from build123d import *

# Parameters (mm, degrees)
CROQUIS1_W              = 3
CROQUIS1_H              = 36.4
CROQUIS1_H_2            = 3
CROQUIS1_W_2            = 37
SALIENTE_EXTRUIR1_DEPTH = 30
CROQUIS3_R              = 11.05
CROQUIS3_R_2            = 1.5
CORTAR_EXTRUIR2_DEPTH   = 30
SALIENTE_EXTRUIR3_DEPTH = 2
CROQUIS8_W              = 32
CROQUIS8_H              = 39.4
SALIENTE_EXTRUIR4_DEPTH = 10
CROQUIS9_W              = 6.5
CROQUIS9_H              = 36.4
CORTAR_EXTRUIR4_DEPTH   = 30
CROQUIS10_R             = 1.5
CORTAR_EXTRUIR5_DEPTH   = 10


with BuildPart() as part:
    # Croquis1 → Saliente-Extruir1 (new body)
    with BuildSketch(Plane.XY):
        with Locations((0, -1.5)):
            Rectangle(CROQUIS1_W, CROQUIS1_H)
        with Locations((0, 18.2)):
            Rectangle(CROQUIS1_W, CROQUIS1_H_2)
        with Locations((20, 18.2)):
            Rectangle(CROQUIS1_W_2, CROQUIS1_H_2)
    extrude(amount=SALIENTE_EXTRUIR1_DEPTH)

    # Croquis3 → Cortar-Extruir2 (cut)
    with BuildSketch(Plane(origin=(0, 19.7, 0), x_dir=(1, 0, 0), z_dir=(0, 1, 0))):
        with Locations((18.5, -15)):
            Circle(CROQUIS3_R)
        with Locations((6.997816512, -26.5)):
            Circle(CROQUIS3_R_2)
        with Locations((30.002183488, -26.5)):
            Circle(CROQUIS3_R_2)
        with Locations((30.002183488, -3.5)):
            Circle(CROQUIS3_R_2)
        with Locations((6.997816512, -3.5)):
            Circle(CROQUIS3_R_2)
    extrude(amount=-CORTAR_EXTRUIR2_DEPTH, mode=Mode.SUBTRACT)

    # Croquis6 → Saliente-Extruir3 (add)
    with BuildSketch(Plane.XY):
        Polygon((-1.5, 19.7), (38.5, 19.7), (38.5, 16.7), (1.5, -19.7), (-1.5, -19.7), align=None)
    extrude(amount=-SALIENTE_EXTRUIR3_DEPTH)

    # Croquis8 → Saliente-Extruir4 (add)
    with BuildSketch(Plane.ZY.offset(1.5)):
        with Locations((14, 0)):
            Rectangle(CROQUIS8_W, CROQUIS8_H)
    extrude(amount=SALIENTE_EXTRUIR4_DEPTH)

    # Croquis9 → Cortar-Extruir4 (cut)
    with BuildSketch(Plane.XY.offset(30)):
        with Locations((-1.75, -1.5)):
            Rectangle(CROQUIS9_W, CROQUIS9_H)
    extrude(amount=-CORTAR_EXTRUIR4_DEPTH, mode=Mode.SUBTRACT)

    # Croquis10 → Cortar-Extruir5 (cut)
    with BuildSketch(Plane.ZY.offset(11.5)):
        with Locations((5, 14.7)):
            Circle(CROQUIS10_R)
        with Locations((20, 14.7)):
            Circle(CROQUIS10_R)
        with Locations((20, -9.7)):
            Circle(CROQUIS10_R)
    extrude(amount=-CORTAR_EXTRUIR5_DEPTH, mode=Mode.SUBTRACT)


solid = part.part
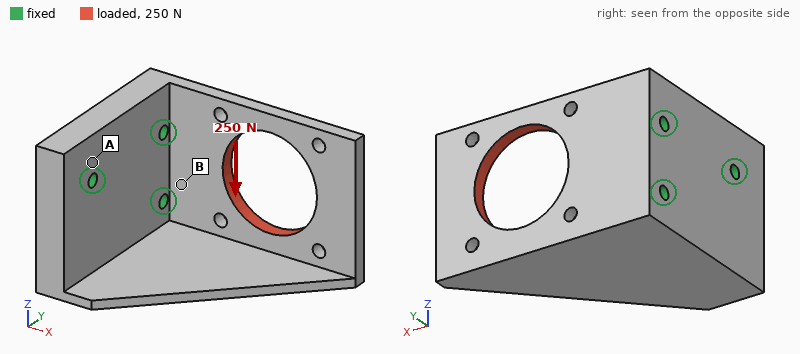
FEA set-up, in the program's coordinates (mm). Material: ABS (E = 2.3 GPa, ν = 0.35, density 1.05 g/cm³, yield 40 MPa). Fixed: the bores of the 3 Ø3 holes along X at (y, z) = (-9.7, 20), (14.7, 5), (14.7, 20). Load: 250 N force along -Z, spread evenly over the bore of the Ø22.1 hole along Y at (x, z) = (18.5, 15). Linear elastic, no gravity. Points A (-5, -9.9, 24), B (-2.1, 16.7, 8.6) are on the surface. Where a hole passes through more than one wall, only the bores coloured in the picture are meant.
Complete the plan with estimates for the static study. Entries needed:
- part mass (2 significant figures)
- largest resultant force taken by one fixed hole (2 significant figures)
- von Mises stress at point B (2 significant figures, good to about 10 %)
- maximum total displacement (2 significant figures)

13 g
350 N
9.5 MPa
0.85 mm
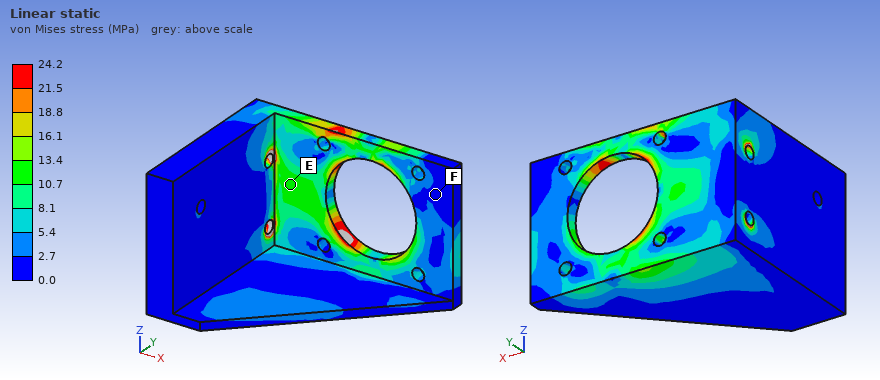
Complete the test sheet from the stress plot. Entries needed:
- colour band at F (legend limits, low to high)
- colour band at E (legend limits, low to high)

0.0 to 2.7 MPa
10.7 to 13.4 MPa
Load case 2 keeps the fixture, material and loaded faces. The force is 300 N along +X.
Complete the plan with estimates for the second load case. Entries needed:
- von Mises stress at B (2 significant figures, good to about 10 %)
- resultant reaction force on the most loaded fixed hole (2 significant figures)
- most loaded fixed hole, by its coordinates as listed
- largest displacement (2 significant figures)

2.3 MPa
190 N
(14.7, 20)
0.22 mm
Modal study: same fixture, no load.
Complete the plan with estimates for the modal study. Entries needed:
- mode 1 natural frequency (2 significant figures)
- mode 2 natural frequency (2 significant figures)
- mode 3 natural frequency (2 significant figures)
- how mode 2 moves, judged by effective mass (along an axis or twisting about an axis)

640 Hz
1500 Hz
1700 Hz
along Z
